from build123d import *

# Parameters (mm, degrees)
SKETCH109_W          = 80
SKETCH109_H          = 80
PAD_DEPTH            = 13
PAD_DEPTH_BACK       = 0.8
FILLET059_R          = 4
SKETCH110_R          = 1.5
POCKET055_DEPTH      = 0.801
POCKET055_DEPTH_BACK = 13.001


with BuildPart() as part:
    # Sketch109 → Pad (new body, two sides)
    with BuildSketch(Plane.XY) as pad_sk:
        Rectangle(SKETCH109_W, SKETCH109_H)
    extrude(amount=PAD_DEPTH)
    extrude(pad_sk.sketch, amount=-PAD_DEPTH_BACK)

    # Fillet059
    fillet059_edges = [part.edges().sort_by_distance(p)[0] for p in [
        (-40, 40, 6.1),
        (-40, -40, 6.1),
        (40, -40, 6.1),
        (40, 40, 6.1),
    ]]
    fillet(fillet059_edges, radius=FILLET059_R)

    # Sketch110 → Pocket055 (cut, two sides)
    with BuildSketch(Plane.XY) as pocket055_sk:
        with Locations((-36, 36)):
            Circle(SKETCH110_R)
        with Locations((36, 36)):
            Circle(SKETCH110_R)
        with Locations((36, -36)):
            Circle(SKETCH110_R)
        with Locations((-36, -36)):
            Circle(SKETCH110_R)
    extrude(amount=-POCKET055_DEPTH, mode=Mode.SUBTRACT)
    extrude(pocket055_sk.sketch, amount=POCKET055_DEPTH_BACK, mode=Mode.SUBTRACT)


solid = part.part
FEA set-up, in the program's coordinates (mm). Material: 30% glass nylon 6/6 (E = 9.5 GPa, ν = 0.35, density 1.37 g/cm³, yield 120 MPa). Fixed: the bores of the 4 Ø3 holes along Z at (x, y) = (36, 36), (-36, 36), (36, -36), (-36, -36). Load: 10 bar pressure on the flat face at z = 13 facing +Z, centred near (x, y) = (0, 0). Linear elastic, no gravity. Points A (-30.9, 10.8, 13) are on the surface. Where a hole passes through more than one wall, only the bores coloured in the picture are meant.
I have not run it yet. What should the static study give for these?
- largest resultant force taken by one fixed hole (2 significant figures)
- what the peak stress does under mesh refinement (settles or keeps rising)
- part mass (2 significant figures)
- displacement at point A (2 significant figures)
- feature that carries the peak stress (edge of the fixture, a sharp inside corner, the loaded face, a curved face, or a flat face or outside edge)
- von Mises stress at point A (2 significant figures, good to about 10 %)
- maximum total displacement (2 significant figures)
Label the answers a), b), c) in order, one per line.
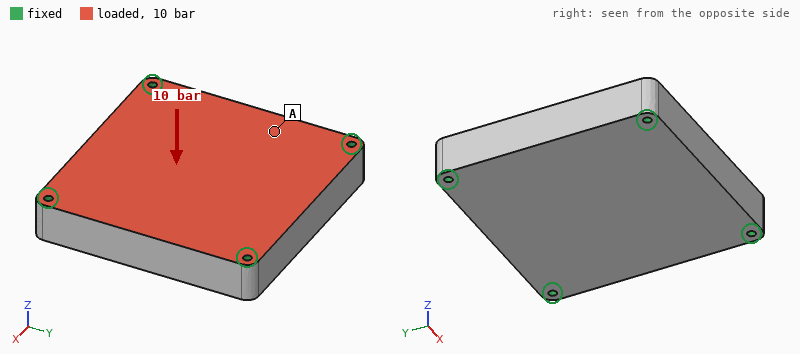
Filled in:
a) 1.6 kN
b) keeps rising
c) 120 g
d) 0.10 mm
e) edge of the fixture
f) 8.9 MPa
g) 0.15 mm
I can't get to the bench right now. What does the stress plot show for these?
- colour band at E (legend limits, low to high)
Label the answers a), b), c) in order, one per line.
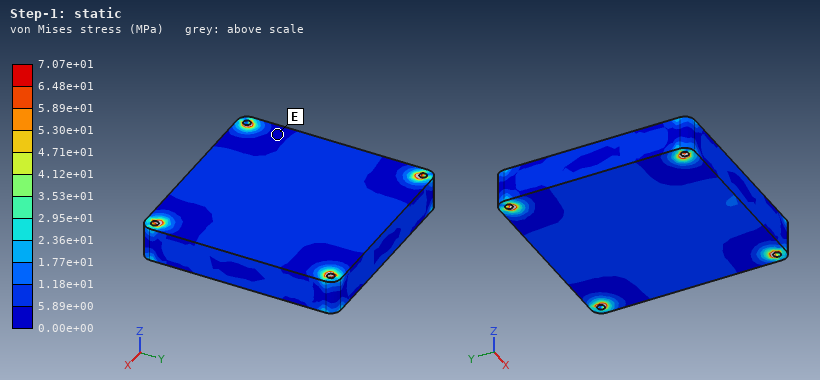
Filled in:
a) 0.00e+00 to 5.89e+00 MPa
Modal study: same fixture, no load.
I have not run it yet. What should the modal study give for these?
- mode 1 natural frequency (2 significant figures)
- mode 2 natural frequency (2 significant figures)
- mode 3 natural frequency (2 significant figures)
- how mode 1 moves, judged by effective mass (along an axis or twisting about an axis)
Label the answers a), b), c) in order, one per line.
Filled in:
a) 3400 Hz
b) 5700 Hz
c) 5700 Hz
d) along Z
